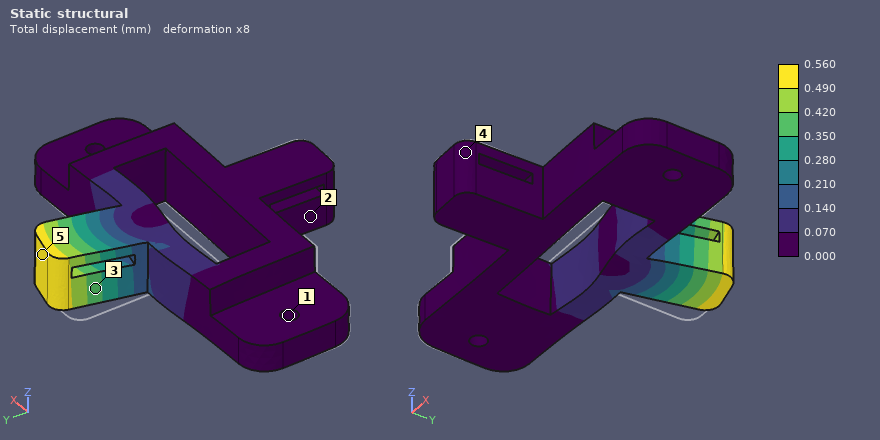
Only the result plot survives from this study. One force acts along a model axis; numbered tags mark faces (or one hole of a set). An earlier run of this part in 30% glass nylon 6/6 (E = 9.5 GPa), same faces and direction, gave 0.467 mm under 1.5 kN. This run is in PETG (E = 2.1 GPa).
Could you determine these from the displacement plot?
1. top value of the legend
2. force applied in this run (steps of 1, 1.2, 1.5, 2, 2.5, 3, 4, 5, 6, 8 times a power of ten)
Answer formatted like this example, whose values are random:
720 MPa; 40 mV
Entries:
0.560 mm; 400 N
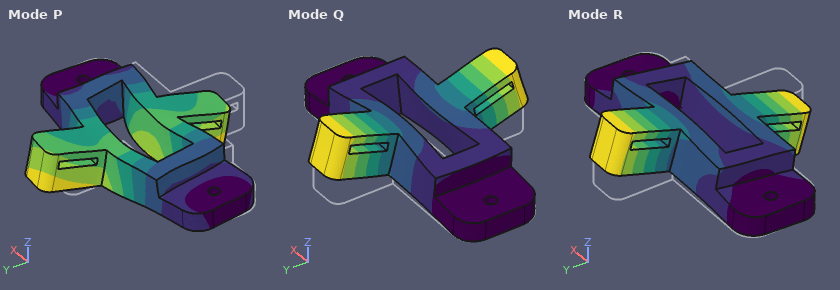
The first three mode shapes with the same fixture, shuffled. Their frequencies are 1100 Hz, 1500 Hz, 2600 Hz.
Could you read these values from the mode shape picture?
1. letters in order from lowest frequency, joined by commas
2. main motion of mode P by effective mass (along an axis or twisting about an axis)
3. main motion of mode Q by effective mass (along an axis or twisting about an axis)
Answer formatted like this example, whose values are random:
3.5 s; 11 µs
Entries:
R, Q, P; along Y; along Z
